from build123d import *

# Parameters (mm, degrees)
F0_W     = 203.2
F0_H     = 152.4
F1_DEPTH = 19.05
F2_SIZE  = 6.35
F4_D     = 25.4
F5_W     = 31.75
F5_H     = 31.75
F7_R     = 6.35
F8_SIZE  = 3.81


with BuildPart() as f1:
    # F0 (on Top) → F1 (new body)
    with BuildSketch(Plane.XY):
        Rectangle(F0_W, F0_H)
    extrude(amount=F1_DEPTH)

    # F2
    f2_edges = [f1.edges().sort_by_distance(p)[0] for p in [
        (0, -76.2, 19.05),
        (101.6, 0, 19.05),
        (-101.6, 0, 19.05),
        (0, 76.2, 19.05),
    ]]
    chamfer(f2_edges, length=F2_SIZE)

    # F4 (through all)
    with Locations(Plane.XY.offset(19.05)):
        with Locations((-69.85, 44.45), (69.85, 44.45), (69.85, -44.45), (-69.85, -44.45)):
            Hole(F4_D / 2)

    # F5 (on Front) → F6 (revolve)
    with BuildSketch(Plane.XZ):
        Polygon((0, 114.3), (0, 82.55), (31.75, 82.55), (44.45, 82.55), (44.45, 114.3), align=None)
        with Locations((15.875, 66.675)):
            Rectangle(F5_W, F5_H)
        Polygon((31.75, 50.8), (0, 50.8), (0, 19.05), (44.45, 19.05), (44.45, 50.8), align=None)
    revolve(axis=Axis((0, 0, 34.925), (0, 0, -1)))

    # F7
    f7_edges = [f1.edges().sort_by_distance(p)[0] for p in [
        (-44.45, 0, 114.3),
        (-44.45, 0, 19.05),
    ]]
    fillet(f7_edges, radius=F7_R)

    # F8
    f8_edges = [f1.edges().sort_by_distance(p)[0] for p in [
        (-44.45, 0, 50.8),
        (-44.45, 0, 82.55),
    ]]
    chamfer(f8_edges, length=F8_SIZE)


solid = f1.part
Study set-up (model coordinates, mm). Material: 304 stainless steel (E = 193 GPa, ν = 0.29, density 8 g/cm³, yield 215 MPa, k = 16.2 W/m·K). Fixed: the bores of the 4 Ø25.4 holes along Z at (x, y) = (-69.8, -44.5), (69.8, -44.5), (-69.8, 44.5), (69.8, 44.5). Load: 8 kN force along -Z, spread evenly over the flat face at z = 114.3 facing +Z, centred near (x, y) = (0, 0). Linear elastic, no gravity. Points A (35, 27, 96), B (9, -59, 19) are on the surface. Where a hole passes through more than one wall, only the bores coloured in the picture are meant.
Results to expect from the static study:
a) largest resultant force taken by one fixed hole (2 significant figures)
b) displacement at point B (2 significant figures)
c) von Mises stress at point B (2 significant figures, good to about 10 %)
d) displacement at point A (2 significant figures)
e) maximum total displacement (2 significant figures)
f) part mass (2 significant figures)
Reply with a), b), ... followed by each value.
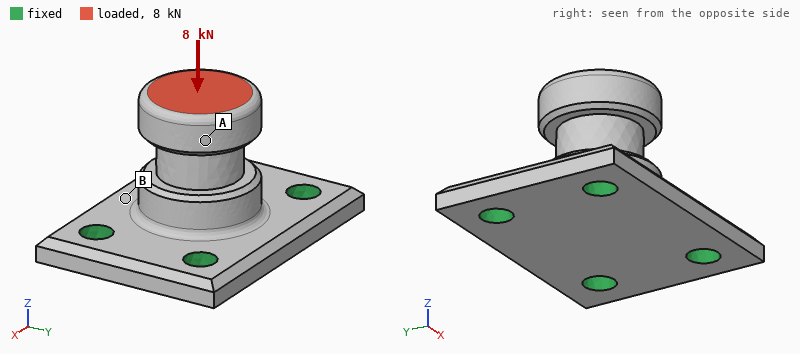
a) 2.2 kN
b) 2.2 µm
c) 2.7 MPa
d) 3.4 µm
e) 3.5 µm
f) 8.2 kg
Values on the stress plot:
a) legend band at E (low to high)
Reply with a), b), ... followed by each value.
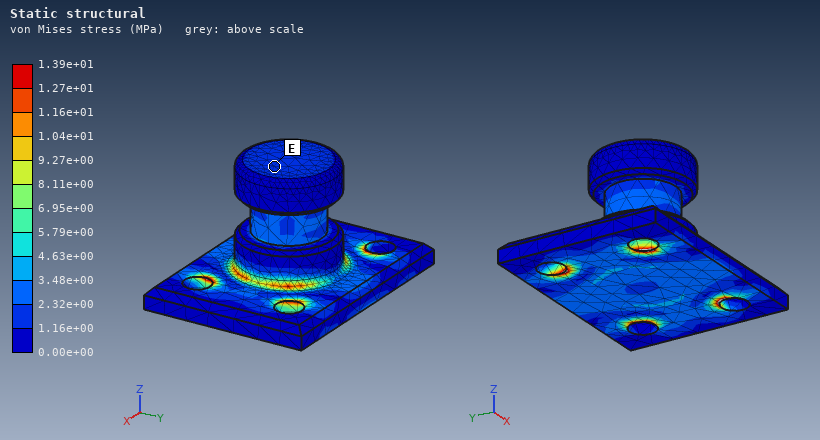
a) 1.16e+00 to 2.32e+00 MPa
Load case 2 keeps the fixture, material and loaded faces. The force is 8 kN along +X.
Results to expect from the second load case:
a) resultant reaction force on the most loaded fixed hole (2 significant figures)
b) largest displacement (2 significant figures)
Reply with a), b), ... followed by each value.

a) 4.5 kN
b) 23 µm
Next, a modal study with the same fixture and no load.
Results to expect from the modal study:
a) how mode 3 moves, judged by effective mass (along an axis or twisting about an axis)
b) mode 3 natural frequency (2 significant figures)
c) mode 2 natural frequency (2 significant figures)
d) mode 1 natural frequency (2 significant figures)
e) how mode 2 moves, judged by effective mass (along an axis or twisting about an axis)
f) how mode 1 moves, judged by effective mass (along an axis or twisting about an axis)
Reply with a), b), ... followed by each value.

a) along Z
b) 3700 Hz
c) 2700 Hz
d) 2100 Hz
e) along X
f) along Y
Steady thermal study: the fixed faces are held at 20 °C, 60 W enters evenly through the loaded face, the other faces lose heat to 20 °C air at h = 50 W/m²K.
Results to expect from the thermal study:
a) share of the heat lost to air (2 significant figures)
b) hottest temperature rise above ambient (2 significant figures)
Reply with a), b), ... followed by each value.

a) 79 %
b) 57 K
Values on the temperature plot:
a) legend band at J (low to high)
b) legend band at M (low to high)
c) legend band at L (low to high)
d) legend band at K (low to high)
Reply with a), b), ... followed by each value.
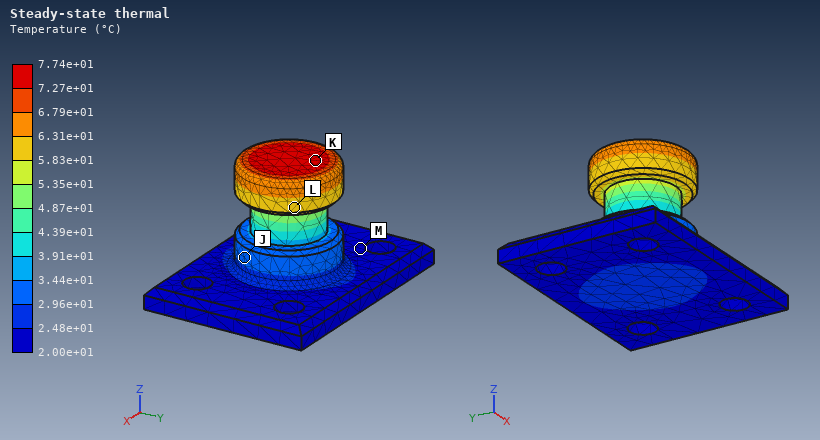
a) 2.96e+01 to 3.44e+01 °C
b) 2.00e+01 to 2.48e+01 °C
c) 5.83e+01 to 6.31e+01 °C
d) 7.27e+01 to 7.74e+01 °C
